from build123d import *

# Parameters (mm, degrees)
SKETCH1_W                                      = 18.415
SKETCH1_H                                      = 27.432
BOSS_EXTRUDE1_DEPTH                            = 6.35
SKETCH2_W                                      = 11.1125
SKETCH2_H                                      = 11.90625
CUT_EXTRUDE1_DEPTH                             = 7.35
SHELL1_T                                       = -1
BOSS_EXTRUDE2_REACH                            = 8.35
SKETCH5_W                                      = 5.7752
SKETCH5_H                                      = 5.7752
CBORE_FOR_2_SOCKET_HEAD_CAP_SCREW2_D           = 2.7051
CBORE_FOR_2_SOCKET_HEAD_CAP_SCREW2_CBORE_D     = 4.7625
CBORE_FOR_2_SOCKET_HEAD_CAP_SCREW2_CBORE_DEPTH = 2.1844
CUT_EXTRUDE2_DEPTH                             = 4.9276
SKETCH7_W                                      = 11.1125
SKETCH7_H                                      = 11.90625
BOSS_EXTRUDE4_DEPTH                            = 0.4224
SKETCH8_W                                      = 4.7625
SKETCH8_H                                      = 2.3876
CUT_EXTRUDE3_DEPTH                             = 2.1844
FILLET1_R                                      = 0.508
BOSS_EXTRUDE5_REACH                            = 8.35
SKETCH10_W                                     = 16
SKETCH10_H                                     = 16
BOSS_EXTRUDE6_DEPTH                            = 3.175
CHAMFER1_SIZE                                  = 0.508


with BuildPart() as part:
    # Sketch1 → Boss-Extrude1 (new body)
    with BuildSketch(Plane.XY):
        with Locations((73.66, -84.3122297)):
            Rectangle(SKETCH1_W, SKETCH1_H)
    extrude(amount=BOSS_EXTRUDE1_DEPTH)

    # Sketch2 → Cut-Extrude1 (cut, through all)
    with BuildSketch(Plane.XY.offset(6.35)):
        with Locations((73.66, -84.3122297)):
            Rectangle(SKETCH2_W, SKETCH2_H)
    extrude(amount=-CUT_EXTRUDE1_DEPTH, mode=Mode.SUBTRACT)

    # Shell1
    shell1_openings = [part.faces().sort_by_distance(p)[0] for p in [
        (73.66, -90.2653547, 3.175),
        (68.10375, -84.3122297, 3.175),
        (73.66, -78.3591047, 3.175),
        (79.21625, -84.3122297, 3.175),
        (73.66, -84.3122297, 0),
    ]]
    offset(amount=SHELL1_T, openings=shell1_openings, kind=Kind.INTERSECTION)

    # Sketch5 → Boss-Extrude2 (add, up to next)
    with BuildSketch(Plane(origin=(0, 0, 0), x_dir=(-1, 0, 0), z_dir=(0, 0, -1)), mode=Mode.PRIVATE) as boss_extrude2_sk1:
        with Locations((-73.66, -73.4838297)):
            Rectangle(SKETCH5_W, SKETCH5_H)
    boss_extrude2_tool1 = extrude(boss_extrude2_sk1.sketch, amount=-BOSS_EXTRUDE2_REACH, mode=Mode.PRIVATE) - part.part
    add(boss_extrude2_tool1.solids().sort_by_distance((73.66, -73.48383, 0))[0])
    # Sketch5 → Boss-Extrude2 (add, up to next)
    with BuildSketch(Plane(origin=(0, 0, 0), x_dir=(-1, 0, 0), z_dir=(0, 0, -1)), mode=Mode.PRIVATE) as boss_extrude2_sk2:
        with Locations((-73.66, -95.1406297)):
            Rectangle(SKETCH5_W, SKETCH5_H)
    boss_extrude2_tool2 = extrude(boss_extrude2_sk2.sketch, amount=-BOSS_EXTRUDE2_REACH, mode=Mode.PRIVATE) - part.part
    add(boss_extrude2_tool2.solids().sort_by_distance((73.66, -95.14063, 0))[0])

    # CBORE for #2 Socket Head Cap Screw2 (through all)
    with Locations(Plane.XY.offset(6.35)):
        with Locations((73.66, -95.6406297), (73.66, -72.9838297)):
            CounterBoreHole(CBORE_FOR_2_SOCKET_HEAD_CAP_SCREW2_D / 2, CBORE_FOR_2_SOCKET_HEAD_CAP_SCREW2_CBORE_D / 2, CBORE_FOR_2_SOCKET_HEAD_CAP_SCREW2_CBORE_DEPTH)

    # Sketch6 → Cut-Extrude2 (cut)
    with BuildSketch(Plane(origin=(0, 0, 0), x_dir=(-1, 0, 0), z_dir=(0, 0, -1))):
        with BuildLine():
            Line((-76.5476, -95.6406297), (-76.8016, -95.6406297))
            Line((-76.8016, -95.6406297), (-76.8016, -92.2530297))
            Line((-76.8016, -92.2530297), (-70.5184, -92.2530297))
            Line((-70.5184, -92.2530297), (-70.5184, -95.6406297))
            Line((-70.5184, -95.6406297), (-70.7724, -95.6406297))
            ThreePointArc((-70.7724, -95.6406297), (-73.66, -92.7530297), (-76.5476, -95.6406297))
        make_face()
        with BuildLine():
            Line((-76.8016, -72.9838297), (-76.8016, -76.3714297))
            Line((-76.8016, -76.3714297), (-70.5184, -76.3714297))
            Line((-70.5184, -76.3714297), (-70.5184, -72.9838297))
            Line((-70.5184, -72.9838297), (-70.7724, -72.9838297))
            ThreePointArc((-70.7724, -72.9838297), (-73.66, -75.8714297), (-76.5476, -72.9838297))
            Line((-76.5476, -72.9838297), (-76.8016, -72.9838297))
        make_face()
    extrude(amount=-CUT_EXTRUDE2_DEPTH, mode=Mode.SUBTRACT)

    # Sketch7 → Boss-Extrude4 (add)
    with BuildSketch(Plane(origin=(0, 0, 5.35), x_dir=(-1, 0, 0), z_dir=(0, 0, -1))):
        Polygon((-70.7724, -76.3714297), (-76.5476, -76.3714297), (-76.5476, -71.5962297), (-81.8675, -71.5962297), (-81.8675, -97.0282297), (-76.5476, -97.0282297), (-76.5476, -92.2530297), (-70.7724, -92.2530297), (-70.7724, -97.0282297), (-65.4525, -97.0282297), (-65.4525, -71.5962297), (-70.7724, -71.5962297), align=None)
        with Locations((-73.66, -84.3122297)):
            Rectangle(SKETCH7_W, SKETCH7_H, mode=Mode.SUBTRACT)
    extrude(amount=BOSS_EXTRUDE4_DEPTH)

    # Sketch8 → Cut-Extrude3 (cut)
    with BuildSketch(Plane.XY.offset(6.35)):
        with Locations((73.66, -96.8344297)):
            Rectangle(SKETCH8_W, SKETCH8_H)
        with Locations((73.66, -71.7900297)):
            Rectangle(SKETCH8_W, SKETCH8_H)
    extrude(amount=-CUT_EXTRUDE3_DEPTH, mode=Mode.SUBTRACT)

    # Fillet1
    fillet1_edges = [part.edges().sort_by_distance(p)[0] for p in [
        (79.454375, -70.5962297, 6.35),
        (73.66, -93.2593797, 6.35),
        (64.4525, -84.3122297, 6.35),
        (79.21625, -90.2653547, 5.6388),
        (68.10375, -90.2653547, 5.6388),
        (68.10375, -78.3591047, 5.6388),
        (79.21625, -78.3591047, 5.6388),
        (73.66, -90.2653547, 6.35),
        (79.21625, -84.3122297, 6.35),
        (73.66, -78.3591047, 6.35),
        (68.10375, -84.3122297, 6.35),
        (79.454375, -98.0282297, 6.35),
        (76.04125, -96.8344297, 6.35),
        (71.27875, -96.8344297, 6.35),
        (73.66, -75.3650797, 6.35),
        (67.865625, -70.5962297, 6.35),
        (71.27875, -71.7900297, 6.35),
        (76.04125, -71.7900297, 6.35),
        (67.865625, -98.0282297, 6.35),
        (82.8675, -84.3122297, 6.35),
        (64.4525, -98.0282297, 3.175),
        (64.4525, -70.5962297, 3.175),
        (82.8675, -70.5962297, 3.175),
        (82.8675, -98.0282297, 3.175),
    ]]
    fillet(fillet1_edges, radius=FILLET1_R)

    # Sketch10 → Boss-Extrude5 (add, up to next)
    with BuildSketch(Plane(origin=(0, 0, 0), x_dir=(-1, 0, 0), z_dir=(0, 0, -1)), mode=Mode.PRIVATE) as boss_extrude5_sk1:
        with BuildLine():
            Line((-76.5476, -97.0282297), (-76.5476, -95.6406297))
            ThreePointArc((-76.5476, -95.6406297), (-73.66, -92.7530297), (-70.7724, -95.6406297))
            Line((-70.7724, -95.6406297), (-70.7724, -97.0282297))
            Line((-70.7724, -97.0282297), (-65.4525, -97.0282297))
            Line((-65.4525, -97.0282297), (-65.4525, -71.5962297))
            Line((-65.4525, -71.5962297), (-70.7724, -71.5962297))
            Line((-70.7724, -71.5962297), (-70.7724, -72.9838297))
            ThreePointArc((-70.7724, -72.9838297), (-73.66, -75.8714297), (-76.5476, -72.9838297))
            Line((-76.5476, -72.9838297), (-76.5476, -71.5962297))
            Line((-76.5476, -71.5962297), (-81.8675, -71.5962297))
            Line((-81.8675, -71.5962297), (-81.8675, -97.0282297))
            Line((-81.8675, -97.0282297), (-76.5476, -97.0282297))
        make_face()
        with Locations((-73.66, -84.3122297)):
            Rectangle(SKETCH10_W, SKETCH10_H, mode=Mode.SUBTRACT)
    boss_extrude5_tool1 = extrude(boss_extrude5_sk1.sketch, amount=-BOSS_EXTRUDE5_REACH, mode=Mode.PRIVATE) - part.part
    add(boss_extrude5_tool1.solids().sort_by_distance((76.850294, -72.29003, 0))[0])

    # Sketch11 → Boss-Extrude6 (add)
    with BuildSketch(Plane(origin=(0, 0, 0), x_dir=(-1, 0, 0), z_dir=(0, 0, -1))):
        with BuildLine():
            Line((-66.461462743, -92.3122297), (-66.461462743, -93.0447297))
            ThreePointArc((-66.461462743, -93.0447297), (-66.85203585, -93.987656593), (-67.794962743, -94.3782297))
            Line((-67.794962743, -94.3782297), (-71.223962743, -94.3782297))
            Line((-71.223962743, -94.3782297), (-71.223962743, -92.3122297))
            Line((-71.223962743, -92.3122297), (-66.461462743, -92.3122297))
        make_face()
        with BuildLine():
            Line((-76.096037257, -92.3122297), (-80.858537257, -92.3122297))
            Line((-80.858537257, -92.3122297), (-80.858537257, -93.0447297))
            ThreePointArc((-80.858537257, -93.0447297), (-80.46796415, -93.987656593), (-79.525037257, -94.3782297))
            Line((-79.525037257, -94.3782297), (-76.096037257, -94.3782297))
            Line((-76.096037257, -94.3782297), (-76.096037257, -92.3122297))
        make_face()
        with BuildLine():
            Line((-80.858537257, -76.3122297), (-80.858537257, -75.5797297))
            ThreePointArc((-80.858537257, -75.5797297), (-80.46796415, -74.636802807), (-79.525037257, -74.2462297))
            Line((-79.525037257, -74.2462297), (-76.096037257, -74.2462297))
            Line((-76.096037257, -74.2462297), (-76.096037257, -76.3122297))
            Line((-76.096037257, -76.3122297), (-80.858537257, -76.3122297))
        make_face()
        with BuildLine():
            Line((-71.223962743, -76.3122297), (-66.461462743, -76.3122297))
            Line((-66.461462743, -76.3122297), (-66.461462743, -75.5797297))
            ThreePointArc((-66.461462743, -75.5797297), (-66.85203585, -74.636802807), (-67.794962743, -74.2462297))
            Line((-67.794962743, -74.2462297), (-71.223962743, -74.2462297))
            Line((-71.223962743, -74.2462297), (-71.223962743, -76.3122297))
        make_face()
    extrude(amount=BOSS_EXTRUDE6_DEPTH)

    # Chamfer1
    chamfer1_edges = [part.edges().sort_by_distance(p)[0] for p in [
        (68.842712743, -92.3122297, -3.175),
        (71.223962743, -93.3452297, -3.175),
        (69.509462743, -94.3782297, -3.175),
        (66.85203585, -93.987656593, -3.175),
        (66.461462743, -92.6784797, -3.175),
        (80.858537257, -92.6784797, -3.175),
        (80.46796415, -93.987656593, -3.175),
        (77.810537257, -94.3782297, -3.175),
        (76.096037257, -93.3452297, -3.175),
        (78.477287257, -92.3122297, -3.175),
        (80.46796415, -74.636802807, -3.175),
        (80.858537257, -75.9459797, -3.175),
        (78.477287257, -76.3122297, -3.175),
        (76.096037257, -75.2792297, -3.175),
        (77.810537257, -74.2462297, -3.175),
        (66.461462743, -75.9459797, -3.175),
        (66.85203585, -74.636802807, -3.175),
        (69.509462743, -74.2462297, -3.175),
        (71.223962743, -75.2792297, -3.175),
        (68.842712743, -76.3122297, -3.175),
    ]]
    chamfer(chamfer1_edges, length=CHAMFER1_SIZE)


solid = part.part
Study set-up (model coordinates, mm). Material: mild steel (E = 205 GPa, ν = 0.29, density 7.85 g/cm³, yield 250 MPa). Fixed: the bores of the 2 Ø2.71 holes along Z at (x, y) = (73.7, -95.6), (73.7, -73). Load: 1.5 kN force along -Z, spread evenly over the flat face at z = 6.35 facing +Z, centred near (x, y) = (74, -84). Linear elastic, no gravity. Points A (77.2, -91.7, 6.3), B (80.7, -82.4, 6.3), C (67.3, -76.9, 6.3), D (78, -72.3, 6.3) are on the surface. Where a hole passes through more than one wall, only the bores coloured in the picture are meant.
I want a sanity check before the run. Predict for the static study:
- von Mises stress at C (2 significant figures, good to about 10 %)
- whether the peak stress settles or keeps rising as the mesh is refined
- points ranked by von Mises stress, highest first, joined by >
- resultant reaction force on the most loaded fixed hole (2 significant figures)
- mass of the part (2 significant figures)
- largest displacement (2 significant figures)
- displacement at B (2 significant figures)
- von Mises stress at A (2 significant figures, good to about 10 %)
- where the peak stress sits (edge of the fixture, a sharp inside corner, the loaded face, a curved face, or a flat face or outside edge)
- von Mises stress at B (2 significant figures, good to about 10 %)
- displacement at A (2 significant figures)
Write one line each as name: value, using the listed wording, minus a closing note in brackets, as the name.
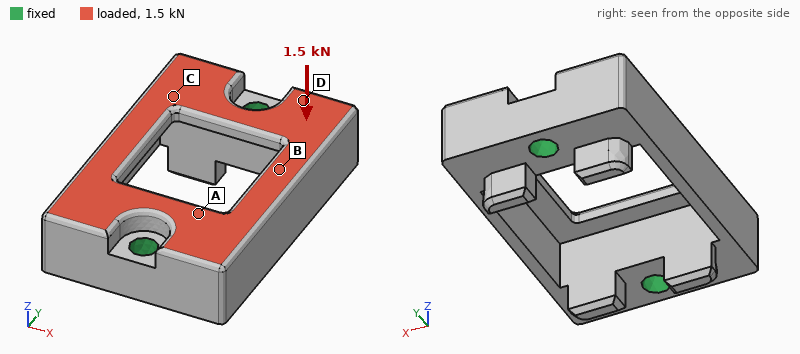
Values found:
von Mises stress at C: 24 MPa
whether the peak stress settles or keeps rising as the mesh is refined: keeps rising
points ranked by von Mises stress, highest first, joined by >: B > A > C > D
resultant reaction force on the most loaded fixed hole: 770 N
mass of the part: 14 g
largest displacement: 8.6 µm
displacement at B: 7.3 µm
von Mises stress at A: 35 MPa
where the peak stress sits: edge of the fixture
von Mises stress at B: 48 MPa
displacement at A: 2.7 µm
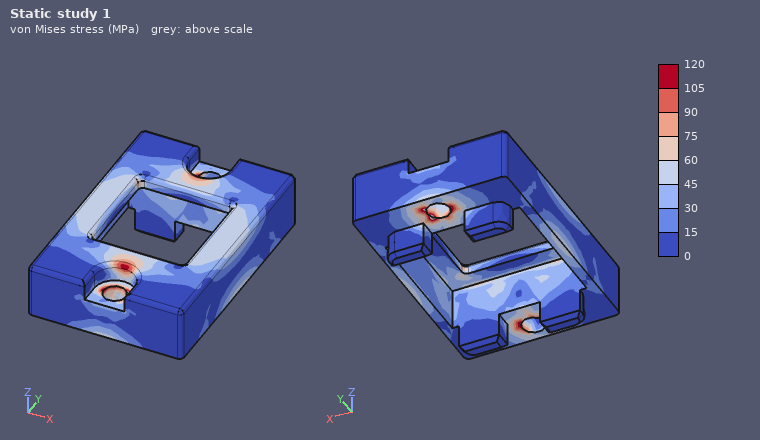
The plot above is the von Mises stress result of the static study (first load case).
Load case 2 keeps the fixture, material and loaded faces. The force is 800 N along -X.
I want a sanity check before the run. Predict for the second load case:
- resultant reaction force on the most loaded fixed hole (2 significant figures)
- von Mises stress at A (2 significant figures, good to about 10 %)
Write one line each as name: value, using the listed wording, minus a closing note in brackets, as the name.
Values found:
resultant reaction force on the most loaded fixed hole: 400 N
von Mises stress at A: 16 MPa
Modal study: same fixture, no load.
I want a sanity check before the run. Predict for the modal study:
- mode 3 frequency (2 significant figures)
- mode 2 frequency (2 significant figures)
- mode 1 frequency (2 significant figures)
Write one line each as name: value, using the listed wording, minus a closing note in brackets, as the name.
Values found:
mode 3 frequency: 28 kHz
mode 2 frequency: 27 kHz
mode 1 frequency: 23 kHz
